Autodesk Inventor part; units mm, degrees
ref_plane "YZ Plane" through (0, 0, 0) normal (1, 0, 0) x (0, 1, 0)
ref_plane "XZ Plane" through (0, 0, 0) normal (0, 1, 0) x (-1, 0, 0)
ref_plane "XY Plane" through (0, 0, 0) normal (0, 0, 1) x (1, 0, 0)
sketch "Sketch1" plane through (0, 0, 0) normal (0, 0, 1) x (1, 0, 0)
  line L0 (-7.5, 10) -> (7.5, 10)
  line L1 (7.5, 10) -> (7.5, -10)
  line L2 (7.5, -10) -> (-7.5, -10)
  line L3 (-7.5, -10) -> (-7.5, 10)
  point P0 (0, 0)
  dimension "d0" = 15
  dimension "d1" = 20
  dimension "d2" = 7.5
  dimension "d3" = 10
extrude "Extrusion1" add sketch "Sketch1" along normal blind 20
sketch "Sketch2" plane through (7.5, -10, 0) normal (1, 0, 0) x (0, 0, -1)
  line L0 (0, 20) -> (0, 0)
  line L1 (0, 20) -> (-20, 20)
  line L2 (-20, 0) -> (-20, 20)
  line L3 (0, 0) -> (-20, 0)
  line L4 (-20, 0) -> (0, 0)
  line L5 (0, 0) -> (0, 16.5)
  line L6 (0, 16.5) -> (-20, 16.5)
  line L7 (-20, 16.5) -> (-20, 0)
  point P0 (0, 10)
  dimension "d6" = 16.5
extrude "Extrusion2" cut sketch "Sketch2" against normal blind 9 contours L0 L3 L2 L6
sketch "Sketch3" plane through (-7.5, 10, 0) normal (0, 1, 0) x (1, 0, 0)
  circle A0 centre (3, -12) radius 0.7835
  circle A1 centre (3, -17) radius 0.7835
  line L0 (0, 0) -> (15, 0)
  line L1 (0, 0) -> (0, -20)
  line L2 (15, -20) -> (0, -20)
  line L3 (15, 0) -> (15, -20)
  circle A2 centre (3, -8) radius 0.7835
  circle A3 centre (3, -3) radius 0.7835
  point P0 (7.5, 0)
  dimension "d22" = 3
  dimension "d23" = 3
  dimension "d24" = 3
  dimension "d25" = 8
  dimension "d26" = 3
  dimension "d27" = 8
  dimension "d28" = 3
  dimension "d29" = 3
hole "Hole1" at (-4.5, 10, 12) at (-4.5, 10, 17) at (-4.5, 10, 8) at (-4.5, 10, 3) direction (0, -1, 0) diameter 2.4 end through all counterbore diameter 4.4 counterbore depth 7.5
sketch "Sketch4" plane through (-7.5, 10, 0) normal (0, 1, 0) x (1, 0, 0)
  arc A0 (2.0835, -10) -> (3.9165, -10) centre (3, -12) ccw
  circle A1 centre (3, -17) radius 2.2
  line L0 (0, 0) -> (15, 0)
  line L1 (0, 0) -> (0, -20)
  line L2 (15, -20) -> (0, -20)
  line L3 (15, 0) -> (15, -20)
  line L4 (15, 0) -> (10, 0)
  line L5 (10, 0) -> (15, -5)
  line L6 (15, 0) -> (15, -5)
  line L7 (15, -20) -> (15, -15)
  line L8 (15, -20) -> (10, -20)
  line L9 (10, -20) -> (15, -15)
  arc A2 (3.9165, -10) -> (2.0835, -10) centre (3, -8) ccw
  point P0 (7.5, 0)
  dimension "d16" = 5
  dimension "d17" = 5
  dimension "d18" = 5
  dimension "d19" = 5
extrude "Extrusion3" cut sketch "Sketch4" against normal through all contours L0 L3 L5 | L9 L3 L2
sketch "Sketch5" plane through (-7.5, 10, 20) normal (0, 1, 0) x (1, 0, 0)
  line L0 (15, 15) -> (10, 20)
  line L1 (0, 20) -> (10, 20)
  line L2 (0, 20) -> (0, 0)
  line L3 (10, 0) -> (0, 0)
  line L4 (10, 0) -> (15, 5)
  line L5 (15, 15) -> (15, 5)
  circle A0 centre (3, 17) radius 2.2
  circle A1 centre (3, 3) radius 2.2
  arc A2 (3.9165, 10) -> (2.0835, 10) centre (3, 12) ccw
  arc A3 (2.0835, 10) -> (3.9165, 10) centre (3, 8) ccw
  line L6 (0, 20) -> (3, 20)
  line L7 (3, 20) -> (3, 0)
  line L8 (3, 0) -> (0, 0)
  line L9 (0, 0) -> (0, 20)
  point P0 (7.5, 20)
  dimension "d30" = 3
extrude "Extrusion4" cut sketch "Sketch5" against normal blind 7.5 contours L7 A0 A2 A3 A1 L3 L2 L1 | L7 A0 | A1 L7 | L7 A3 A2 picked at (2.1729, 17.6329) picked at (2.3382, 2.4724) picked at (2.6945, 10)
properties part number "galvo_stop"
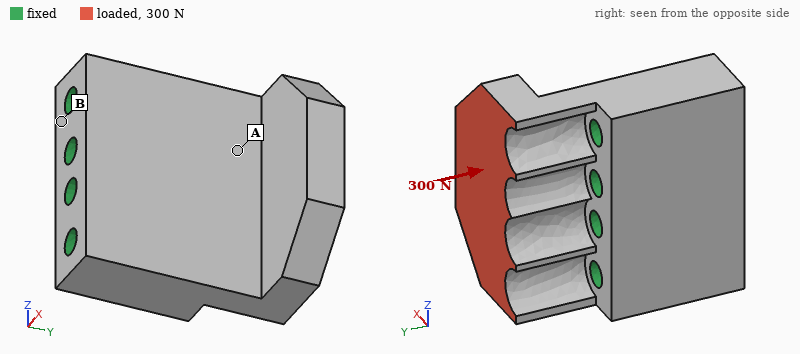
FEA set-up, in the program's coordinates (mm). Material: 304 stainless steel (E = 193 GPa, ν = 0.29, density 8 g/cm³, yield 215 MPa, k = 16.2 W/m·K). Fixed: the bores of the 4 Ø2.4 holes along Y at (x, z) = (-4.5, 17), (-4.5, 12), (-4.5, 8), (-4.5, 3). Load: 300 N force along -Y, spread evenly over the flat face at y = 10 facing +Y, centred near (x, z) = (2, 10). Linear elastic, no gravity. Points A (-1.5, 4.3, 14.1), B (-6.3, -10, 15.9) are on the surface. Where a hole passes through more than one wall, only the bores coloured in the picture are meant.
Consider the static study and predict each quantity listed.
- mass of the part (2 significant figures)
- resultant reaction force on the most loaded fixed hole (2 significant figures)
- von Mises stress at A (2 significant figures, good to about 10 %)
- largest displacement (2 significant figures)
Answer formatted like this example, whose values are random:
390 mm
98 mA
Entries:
16 g
91 N
82 MPa
33 µm
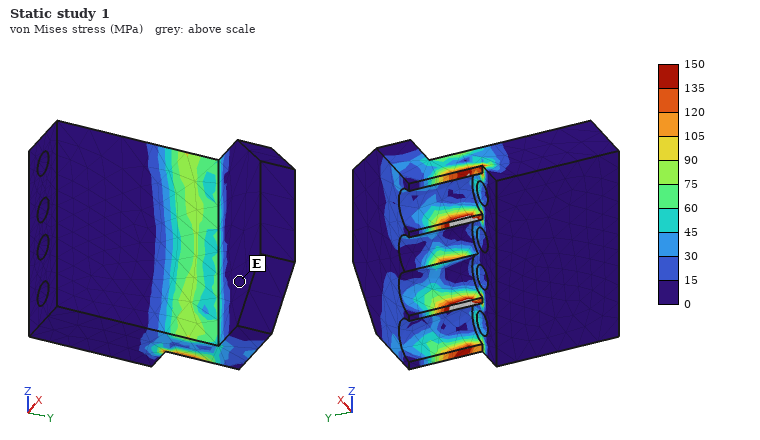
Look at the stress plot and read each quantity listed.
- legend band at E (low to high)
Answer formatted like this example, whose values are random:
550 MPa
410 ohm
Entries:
0 to 15 MPa
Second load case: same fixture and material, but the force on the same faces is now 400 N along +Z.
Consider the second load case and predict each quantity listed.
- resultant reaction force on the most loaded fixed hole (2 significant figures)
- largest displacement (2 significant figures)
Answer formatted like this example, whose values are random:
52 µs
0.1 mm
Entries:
270 N
5.5 µm
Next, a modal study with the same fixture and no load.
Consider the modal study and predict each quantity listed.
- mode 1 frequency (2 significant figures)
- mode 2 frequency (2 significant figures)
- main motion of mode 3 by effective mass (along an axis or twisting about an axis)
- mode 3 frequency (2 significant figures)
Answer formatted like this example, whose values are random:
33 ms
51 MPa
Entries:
7200 Hz
16 kHz
along X
24 kHz
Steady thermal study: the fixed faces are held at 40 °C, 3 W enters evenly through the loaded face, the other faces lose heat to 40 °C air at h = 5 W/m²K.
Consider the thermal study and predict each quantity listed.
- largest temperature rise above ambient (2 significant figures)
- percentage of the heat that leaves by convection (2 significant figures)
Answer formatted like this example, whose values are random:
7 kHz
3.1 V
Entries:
49 K
3.5 %
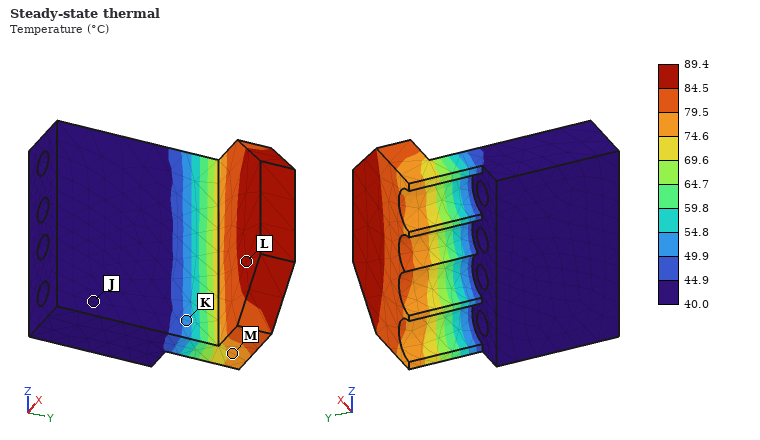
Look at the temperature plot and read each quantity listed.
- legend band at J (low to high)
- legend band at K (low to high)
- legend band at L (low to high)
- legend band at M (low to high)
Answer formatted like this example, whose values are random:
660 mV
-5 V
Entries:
40.0 to 44.9 °C
49.9 to 54.8 °C
84.5 to 89.4 °C
74.6 to 79.5 °C
